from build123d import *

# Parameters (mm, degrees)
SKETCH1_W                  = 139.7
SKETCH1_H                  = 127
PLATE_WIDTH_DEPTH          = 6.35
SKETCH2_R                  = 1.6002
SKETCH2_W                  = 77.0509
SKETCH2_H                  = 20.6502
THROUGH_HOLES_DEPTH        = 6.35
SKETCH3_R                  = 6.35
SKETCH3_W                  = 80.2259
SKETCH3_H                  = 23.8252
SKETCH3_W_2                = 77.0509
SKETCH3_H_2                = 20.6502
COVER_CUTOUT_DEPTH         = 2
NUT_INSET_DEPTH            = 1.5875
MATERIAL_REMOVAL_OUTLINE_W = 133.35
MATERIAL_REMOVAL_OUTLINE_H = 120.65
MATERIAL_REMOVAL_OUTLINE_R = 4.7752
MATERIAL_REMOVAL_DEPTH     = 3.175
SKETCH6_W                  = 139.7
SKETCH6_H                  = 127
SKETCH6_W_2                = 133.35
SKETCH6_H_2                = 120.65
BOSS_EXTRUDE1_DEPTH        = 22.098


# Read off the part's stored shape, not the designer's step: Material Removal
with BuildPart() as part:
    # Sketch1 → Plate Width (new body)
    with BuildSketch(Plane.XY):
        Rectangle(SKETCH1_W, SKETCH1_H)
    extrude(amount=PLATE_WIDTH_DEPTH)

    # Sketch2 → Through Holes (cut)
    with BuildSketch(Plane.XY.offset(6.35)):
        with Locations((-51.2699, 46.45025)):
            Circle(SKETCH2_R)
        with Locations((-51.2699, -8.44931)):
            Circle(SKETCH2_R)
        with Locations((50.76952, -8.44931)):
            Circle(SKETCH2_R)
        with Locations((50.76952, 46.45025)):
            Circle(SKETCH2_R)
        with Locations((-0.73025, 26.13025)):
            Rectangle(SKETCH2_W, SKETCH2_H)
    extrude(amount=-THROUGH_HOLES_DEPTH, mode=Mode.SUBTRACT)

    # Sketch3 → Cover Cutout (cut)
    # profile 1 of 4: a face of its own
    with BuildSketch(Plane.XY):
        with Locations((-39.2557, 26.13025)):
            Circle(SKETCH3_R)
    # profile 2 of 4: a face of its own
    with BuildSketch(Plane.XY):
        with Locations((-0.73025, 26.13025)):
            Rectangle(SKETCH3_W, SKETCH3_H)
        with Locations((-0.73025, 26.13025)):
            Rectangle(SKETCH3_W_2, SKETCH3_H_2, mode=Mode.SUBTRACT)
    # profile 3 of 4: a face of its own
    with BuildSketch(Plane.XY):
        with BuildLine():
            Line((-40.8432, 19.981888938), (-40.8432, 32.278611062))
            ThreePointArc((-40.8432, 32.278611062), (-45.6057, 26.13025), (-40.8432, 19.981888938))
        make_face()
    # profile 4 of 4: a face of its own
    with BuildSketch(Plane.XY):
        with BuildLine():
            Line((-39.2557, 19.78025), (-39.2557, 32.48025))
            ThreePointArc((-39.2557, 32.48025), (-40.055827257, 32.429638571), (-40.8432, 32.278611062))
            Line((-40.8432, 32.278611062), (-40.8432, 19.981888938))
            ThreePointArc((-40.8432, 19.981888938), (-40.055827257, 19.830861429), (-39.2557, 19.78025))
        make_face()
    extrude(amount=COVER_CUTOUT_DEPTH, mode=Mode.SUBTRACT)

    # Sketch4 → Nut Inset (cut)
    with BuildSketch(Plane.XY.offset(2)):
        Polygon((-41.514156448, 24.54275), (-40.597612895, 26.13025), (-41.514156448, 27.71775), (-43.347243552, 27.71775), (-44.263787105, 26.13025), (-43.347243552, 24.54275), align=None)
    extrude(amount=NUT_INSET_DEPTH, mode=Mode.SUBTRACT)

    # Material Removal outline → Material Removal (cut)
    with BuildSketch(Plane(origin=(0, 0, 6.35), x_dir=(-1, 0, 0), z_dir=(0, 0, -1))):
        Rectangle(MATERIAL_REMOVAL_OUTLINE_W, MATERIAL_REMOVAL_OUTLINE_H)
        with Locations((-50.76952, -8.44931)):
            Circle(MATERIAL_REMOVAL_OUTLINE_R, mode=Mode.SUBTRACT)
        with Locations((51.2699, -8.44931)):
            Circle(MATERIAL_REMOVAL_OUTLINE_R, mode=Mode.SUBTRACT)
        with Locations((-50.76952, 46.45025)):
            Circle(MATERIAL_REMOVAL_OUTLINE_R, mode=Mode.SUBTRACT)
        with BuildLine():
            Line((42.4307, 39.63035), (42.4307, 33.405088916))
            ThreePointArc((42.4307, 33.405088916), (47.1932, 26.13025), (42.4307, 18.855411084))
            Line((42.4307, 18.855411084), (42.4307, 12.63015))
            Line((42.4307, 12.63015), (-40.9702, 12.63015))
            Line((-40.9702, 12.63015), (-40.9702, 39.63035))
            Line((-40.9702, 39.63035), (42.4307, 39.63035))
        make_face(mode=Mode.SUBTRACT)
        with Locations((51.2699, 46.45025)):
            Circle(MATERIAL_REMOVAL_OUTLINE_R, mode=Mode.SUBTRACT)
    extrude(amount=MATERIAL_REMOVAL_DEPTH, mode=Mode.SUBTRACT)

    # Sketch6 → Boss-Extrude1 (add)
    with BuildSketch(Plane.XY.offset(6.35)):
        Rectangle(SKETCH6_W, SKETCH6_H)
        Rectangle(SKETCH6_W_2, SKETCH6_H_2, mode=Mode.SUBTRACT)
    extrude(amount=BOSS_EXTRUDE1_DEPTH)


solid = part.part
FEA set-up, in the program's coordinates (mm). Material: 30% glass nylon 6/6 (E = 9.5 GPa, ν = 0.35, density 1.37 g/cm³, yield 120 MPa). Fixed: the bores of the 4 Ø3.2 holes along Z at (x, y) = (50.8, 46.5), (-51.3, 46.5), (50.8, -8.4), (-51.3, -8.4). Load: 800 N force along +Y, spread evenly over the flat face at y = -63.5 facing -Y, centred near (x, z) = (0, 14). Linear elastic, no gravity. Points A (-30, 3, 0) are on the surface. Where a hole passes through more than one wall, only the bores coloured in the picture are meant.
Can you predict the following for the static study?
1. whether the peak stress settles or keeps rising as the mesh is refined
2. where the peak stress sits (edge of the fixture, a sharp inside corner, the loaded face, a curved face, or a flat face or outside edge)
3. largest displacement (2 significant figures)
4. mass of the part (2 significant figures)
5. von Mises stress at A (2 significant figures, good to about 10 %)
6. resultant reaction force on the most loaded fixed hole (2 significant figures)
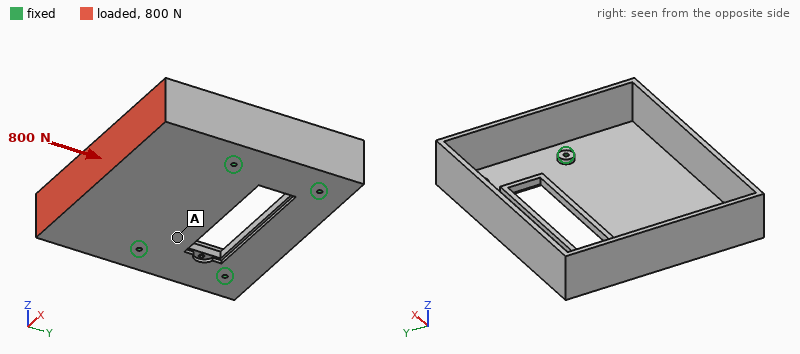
keeps rising
edge of the fixture
1.4 mm
130 g
3.5 MPa
300 N
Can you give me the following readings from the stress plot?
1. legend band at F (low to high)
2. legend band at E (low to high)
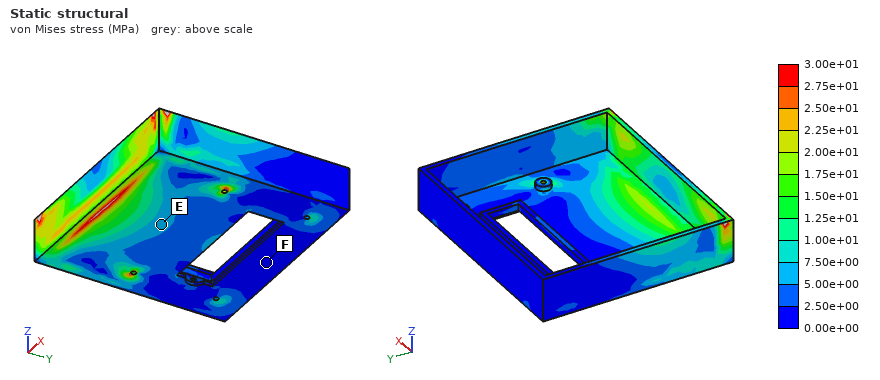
0.00e+00 to 2.50e+00 MPa
5.00e+00 to 7.50e+00 MPa
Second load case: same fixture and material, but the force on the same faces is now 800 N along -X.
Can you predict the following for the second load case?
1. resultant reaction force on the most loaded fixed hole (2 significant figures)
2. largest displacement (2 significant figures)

560 N
0.47 mm
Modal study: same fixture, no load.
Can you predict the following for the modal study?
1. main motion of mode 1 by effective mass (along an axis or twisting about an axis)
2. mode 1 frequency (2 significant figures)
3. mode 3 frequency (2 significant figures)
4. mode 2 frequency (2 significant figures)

along Z
580 Hz
970 Hz
720 Hz
